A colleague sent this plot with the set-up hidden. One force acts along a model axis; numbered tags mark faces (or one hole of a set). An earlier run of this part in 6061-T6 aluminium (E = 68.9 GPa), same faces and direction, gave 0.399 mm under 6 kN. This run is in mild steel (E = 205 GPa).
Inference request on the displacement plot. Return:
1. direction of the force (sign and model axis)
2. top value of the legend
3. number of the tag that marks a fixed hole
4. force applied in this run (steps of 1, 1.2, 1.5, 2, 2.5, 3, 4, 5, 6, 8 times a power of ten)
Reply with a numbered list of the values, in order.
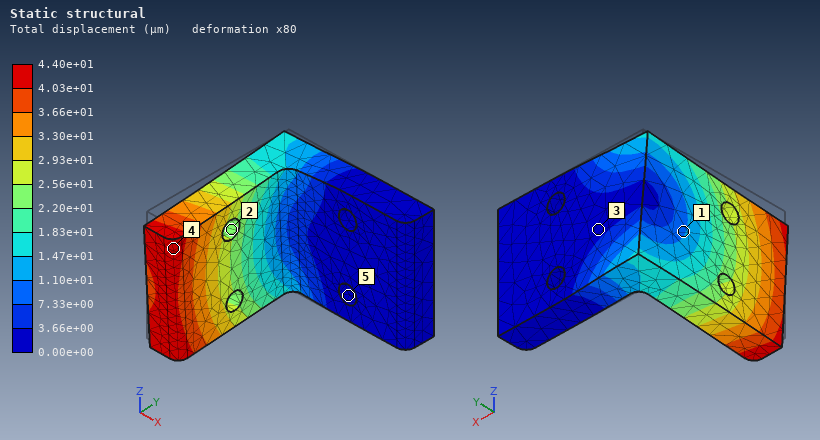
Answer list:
1. -Z
2. 4.40e+01 µm
3. 5
4. 2 kN
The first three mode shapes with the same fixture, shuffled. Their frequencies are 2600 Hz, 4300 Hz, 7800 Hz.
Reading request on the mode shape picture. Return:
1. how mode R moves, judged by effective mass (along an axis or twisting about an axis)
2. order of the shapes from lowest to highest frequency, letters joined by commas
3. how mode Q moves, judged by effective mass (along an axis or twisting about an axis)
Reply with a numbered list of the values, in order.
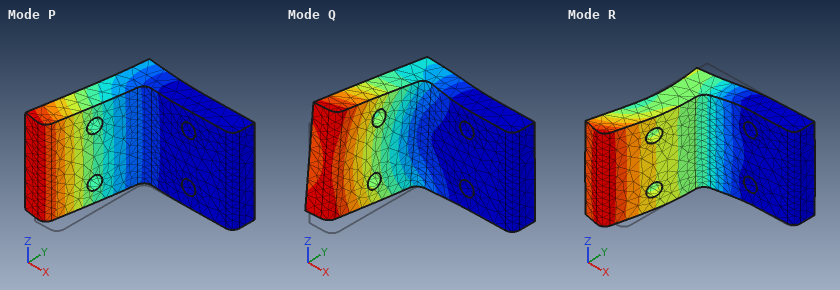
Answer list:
1. along Y
2. P, Q, R
3. along Z
